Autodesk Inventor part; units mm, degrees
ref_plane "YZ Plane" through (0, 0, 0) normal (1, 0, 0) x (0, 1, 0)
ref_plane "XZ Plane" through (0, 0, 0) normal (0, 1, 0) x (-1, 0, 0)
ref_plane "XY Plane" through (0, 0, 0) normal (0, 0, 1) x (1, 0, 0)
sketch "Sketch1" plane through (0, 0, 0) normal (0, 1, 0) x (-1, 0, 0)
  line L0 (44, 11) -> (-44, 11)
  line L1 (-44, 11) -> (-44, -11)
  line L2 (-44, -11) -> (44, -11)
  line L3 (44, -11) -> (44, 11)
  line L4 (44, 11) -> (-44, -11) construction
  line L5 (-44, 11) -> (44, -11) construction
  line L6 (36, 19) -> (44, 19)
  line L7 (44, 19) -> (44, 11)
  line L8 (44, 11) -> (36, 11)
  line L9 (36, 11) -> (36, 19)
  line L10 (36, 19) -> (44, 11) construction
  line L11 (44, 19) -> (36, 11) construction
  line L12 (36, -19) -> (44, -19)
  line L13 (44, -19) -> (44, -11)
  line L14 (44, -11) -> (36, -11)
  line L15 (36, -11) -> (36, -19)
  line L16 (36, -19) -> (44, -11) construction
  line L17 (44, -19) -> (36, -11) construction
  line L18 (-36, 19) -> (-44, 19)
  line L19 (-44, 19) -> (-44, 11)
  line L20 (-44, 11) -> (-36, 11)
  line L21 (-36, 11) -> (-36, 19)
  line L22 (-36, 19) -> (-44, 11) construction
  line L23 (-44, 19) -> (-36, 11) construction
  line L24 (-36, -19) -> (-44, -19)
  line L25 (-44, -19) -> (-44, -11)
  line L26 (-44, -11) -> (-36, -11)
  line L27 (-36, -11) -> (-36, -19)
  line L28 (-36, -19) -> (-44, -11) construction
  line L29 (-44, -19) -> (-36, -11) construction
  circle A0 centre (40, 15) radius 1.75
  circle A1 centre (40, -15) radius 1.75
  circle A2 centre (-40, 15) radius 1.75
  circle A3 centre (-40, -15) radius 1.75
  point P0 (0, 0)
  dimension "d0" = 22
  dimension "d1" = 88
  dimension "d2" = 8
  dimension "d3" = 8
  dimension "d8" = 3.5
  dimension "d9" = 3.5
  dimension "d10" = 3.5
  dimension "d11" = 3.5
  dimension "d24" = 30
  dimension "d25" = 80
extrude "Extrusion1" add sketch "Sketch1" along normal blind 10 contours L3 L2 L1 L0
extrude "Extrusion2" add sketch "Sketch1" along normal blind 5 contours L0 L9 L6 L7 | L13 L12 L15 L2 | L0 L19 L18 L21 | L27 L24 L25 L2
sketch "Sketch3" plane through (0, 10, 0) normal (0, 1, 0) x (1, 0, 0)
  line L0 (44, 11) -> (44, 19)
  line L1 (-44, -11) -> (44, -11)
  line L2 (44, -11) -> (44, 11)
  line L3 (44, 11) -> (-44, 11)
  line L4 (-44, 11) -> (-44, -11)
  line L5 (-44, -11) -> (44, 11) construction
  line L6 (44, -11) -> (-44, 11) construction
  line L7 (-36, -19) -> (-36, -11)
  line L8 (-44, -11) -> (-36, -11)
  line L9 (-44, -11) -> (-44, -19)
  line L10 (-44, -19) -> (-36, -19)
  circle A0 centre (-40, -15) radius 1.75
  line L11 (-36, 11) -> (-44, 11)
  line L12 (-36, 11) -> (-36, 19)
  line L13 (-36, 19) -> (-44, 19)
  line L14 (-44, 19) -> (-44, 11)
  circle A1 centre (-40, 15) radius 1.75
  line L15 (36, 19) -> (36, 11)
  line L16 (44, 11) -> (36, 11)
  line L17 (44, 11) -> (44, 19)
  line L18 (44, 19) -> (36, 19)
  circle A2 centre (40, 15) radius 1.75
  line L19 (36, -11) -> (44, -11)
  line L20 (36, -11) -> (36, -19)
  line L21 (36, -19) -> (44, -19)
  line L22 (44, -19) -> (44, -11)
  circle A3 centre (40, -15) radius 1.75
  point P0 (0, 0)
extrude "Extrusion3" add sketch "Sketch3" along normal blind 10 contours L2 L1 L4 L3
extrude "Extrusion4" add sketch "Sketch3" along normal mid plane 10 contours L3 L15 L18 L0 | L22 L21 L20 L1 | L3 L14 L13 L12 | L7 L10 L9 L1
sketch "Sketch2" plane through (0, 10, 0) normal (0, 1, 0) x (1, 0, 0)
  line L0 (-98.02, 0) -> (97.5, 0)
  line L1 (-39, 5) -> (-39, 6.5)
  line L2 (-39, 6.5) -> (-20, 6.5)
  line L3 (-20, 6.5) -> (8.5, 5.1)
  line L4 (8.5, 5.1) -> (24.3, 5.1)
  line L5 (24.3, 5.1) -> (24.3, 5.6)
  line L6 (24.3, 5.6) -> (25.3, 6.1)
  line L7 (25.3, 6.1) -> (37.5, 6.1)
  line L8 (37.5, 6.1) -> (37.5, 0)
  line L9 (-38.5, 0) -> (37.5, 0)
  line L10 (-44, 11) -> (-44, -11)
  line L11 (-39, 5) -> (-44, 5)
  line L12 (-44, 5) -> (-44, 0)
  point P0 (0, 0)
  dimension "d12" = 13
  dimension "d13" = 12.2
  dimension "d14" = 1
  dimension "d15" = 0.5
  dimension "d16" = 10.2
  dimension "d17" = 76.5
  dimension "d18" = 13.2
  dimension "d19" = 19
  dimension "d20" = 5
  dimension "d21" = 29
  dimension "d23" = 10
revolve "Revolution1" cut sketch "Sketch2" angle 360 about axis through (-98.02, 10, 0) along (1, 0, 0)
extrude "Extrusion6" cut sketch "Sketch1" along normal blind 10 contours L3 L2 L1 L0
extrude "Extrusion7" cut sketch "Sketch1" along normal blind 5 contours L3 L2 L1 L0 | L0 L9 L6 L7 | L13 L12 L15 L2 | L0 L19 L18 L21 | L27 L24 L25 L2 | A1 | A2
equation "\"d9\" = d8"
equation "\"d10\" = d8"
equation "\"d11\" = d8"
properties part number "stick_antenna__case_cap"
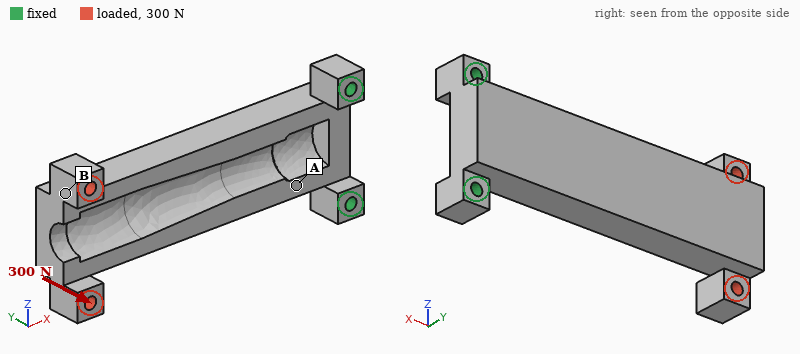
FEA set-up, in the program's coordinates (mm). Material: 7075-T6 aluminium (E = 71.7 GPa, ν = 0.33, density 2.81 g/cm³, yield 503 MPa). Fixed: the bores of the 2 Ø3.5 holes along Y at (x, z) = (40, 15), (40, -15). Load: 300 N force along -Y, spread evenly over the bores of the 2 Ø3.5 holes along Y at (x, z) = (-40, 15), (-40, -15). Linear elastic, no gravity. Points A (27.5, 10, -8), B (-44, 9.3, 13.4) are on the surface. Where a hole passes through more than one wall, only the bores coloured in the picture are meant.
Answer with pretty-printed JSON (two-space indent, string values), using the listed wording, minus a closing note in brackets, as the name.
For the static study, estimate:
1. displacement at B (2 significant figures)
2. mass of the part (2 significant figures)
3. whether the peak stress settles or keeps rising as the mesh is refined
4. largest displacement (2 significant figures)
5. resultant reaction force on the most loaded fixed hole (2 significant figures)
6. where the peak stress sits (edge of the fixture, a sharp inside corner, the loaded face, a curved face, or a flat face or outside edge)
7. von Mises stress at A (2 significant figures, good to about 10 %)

{
  "displacement at B": "1.1 mm",
  "mass of the part": "48 g",
  "whether the peak stress settles or keeps rising as the mesh is refined": "keeps rising",
  "largest displacement": "1.1 mm",
  "resultant reaction force on the most loaded fixed hole": "270 N",
  "where the peak stress sits": "a sharp inside corner",
  "von Mises stress at A": "96 MPa"
}
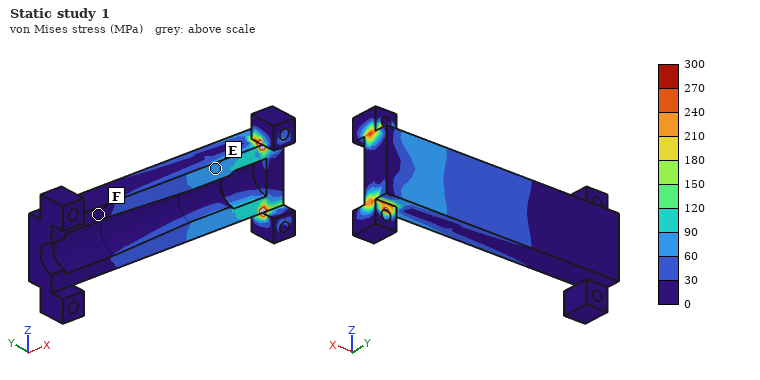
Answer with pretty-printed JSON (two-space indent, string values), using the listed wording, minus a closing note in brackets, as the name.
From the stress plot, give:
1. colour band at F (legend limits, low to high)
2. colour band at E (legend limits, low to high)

{
  "colour band at F": "0 to 30 MPa",
  "colour band at E": "60 to 90 MPa"
}
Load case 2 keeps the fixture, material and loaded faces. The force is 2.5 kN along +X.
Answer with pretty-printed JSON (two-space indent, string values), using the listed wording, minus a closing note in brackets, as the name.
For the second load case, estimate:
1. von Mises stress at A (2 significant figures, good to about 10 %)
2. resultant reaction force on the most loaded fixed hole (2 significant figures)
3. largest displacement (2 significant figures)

{
  "von Mises stress at A": "85 MPa",
  "resultant reaction force on the most loaded fixed hole": "1.3 kN",
  "largest displacement": "0.66 mm"
}
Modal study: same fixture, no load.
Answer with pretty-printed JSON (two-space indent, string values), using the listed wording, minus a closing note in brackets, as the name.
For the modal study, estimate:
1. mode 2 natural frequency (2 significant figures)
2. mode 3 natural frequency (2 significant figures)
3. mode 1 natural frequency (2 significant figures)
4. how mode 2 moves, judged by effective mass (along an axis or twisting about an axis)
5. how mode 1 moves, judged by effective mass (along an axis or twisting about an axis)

{
  "mode 2 natural frequency": "1900 Hz",
  "mode 3 natural frequency": "3300 Hz",
  "mode 1 natural frequency": "700 Hz",
  "how mode 2 moves, judged by effective mass": "along Z",
  "how mode 1 moves, judged by effective mass": "along Y"
}
